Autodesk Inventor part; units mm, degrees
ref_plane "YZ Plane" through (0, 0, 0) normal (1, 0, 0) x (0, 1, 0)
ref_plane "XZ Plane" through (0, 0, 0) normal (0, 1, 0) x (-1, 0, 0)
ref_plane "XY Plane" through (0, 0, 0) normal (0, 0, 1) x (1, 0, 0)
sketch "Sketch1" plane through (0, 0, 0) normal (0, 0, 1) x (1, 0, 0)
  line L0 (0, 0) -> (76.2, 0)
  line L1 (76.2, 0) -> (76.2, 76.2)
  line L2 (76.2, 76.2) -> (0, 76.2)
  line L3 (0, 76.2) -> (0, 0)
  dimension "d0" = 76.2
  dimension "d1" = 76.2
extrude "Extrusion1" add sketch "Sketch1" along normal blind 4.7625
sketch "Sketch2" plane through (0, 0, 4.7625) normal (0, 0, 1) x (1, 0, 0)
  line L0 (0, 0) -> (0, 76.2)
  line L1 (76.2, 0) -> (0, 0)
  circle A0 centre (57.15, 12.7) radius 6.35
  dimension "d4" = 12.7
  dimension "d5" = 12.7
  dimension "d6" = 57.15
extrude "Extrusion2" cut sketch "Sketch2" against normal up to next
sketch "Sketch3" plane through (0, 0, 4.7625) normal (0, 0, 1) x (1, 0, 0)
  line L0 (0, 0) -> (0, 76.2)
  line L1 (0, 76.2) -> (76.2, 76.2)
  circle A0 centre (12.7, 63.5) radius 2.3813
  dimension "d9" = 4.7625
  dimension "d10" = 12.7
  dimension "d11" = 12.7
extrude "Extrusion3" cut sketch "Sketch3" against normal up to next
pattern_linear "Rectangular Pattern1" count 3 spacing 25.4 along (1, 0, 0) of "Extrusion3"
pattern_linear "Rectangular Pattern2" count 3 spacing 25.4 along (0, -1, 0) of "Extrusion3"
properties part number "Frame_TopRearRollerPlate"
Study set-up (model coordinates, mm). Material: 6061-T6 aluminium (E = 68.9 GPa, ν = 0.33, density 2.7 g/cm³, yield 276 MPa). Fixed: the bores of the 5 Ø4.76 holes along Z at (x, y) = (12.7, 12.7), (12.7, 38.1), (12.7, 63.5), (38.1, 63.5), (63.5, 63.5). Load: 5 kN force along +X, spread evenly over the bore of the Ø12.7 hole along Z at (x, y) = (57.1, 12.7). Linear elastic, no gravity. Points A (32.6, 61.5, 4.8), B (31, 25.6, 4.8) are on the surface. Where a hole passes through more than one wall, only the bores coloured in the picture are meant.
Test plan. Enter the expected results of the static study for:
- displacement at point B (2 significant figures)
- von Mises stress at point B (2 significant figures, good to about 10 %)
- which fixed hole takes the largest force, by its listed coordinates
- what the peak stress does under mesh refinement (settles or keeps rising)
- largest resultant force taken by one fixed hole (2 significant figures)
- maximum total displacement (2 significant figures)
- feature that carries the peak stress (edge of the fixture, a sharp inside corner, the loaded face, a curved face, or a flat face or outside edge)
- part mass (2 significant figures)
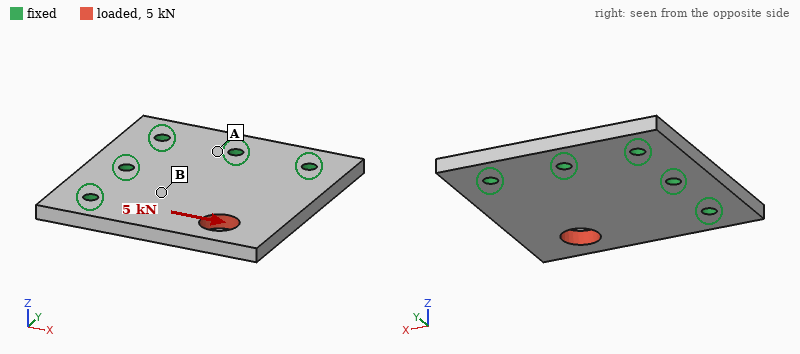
6.1 µm
19 MPa
(12.7, 12.7)
keeps rising
3.1 kN
31 µm
edge of the fixture
72 g
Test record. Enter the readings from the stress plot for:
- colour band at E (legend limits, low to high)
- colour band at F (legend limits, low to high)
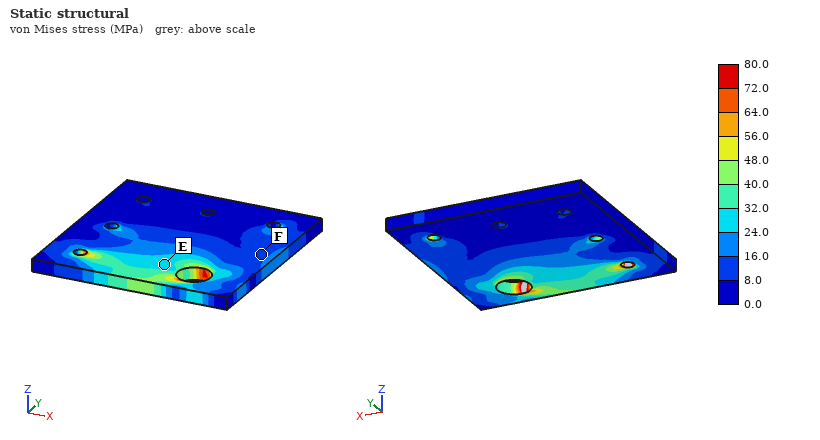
24.0 to 32.0 MPa
8.0 to 16.0 MPa
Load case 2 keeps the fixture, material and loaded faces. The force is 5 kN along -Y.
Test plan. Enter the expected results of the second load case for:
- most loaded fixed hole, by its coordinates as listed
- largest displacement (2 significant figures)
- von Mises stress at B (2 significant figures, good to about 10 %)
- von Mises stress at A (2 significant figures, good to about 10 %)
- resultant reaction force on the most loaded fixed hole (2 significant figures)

(63.5, 63.5)
32 µm
14 MPa
6.3 MPa
2.7 kN
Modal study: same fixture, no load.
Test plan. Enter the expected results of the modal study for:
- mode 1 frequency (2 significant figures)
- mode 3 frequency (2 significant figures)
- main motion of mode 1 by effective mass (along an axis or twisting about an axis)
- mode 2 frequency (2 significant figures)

2000 Hz
6900 Hz
along Z
6100 Hz
